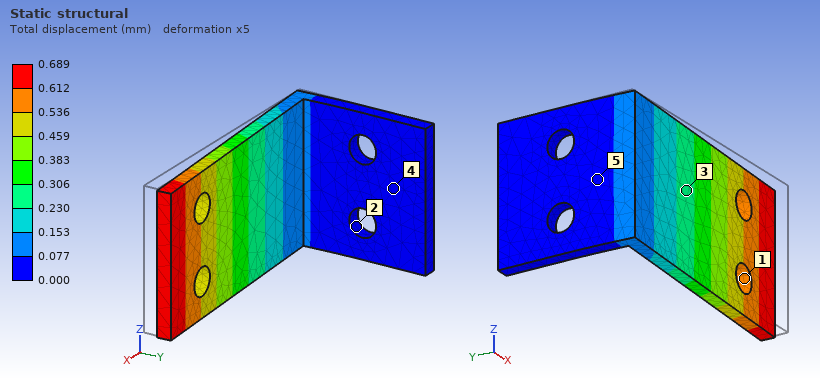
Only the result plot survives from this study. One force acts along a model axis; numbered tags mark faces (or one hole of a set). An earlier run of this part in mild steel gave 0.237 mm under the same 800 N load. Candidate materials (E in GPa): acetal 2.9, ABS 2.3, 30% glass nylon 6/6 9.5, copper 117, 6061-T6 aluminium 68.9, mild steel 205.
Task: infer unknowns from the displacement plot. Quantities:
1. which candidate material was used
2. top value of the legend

6061-T6 aluminium
0.689 mm
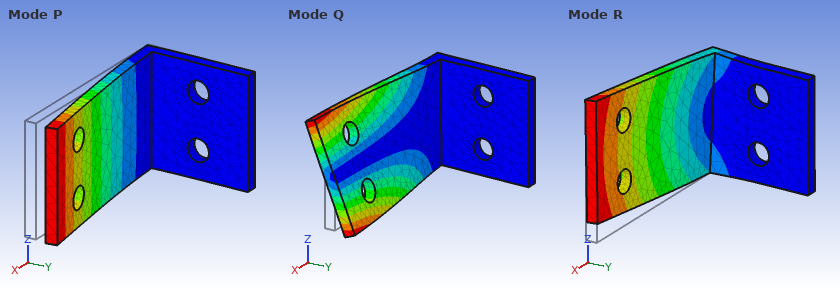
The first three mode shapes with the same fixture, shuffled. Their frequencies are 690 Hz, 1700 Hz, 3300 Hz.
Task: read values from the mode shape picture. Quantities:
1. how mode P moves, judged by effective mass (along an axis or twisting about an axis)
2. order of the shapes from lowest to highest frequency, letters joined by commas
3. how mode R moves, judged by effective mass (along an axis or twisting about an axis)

along Y
P, R, Q
along Z
